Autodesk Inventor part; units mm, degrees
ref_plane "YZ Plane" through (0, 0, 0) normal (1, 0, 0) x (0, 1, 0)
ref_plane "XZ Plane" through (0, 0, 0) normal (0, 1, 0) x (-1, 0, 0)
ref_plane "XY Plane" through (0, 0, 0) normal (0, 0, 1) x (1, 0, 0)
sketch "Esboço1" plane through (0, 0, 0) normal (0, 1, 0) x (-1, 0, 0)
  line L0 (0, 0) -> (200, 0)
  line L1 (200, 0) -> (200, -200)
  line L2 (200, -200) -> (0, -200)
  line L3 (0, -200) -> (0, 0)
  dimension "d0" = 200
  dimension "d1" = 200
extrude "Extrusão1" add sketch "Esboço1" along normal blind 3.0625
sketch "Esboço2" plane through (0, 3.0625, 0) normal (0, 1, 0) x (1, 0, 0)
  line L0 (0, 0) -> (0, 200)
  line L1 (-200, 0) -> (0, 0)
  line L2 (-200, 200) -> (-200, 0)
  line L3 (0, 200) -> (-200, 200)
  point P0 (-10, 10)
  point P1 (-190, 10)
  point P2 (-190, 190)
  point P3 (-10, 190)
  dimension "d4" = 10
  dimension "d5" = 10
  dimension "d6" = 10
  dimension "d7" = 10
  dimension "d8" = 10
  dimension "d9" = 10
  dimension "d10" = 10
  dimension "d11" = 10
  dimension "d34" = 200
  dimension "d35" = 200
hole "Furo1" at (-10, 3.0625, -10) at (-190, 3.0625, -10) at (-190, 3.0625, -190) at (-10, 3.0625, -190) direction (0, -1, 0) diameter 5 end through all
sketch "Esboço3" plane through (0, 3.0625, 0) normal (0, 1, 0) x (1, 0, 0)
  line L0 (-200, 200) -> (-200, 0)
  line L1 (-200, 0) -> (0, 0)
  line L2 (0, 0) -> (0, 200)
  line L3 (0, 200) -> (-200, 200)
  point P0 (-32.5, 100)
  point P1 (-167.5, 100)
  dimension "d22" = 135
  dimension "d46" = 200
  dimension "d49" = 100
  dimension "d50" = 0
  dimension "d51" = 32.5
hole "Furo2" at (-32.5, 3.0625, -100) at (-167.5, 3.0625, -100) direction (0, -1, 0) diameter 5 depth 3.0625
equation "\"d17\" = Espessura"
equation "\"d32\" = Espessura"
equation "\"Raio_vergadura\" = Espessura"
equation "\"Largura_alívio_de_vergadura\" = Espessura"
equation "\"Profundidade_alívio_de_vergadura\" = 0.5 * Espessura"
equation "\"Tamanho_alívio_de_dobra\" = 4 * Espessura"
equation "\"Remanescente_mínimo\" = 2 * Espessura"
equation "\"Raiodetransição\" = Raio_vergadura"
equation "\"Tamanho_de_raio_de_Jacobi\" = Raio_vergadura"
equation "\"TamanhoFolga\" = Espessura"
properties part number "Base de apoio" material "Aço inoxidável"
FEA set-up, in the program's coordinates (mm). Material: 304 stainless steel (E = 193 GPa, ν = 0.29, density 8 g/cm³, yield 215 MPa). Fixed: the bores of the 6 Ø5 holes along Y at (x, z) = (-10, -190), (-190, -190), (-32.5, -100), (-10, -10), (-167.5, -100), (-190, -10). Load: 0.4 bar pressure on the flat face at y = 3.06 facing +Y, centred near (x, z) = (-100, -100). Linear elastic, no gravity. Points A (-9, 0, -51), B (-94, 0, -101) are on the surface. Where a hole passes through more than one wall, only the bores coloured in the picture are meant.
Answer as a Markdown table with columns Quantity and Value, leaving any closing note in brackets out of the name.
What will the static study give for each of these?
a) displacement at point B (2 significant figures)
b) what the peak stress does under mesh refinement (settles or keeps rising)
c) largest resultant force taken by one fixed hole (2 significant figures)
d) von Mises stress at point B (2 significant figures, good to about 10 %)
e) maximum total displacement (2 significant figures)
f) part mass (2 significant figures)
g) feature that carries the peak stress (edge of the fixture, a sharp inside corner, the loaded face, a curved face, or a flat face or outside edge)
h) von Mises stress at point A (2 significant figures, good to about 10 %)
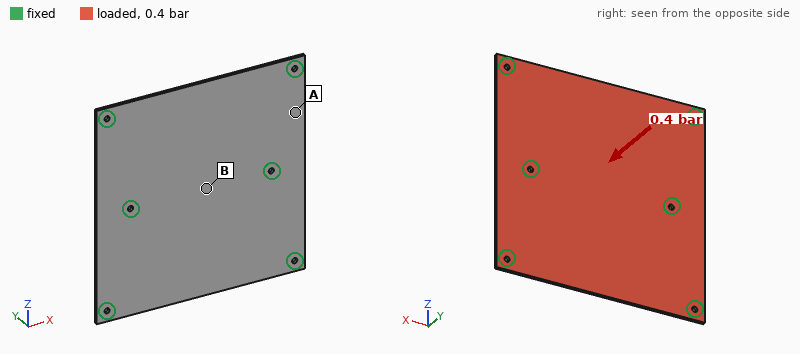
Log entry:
| Quantity | Value |
|---|---|
| displacement at point B | 0.14 mm |
| what the peak stress does under mesh refinement | keeps rising |
| largest resultant force taken by one fixed hole | 430 N |
| von Mises stress at point B | 32 MPa |
| maximum total displacement | 0.25 mm |
| part mass | 980 g |
| feature that carries the peak stress | edge of the fixture |
| von Mises stress at point A | 10 MPa |
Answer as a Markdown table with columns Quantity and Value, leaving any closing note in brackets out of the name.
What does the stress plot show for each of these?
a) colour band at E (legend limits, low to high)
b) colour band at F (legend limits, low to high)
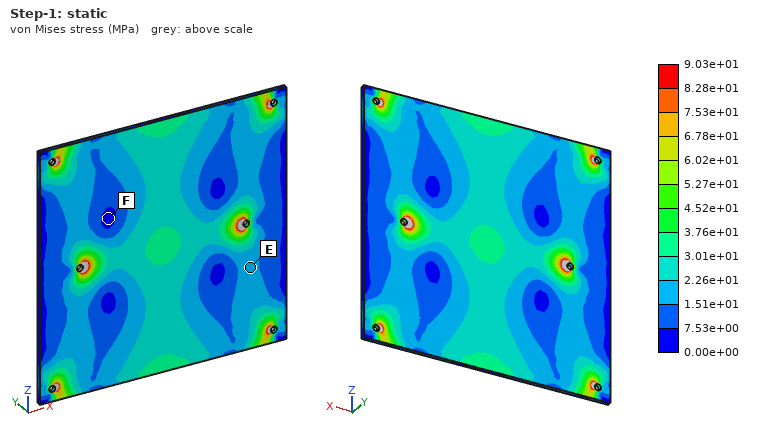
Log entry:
| Quantity | Value |
|---|---|
| colour band at E | 1.51e+01 to 2.26e+01 MPa |
| colour band at F | 0.00e+00 to 7.53e+00 MPa |
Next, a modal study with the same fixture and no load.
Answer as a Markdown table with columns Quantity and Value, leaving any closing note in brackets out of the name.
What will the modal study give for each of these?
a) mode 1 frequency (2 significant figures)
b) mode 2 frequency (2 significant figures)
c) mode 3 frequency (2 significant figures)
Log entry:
| Quantity | Value |
|---|---|
| mode 1 frequency | 510 Hz |
| mode 2 frequency | 530 Hz |
| mode 3 frequency | 1000 Hz |
